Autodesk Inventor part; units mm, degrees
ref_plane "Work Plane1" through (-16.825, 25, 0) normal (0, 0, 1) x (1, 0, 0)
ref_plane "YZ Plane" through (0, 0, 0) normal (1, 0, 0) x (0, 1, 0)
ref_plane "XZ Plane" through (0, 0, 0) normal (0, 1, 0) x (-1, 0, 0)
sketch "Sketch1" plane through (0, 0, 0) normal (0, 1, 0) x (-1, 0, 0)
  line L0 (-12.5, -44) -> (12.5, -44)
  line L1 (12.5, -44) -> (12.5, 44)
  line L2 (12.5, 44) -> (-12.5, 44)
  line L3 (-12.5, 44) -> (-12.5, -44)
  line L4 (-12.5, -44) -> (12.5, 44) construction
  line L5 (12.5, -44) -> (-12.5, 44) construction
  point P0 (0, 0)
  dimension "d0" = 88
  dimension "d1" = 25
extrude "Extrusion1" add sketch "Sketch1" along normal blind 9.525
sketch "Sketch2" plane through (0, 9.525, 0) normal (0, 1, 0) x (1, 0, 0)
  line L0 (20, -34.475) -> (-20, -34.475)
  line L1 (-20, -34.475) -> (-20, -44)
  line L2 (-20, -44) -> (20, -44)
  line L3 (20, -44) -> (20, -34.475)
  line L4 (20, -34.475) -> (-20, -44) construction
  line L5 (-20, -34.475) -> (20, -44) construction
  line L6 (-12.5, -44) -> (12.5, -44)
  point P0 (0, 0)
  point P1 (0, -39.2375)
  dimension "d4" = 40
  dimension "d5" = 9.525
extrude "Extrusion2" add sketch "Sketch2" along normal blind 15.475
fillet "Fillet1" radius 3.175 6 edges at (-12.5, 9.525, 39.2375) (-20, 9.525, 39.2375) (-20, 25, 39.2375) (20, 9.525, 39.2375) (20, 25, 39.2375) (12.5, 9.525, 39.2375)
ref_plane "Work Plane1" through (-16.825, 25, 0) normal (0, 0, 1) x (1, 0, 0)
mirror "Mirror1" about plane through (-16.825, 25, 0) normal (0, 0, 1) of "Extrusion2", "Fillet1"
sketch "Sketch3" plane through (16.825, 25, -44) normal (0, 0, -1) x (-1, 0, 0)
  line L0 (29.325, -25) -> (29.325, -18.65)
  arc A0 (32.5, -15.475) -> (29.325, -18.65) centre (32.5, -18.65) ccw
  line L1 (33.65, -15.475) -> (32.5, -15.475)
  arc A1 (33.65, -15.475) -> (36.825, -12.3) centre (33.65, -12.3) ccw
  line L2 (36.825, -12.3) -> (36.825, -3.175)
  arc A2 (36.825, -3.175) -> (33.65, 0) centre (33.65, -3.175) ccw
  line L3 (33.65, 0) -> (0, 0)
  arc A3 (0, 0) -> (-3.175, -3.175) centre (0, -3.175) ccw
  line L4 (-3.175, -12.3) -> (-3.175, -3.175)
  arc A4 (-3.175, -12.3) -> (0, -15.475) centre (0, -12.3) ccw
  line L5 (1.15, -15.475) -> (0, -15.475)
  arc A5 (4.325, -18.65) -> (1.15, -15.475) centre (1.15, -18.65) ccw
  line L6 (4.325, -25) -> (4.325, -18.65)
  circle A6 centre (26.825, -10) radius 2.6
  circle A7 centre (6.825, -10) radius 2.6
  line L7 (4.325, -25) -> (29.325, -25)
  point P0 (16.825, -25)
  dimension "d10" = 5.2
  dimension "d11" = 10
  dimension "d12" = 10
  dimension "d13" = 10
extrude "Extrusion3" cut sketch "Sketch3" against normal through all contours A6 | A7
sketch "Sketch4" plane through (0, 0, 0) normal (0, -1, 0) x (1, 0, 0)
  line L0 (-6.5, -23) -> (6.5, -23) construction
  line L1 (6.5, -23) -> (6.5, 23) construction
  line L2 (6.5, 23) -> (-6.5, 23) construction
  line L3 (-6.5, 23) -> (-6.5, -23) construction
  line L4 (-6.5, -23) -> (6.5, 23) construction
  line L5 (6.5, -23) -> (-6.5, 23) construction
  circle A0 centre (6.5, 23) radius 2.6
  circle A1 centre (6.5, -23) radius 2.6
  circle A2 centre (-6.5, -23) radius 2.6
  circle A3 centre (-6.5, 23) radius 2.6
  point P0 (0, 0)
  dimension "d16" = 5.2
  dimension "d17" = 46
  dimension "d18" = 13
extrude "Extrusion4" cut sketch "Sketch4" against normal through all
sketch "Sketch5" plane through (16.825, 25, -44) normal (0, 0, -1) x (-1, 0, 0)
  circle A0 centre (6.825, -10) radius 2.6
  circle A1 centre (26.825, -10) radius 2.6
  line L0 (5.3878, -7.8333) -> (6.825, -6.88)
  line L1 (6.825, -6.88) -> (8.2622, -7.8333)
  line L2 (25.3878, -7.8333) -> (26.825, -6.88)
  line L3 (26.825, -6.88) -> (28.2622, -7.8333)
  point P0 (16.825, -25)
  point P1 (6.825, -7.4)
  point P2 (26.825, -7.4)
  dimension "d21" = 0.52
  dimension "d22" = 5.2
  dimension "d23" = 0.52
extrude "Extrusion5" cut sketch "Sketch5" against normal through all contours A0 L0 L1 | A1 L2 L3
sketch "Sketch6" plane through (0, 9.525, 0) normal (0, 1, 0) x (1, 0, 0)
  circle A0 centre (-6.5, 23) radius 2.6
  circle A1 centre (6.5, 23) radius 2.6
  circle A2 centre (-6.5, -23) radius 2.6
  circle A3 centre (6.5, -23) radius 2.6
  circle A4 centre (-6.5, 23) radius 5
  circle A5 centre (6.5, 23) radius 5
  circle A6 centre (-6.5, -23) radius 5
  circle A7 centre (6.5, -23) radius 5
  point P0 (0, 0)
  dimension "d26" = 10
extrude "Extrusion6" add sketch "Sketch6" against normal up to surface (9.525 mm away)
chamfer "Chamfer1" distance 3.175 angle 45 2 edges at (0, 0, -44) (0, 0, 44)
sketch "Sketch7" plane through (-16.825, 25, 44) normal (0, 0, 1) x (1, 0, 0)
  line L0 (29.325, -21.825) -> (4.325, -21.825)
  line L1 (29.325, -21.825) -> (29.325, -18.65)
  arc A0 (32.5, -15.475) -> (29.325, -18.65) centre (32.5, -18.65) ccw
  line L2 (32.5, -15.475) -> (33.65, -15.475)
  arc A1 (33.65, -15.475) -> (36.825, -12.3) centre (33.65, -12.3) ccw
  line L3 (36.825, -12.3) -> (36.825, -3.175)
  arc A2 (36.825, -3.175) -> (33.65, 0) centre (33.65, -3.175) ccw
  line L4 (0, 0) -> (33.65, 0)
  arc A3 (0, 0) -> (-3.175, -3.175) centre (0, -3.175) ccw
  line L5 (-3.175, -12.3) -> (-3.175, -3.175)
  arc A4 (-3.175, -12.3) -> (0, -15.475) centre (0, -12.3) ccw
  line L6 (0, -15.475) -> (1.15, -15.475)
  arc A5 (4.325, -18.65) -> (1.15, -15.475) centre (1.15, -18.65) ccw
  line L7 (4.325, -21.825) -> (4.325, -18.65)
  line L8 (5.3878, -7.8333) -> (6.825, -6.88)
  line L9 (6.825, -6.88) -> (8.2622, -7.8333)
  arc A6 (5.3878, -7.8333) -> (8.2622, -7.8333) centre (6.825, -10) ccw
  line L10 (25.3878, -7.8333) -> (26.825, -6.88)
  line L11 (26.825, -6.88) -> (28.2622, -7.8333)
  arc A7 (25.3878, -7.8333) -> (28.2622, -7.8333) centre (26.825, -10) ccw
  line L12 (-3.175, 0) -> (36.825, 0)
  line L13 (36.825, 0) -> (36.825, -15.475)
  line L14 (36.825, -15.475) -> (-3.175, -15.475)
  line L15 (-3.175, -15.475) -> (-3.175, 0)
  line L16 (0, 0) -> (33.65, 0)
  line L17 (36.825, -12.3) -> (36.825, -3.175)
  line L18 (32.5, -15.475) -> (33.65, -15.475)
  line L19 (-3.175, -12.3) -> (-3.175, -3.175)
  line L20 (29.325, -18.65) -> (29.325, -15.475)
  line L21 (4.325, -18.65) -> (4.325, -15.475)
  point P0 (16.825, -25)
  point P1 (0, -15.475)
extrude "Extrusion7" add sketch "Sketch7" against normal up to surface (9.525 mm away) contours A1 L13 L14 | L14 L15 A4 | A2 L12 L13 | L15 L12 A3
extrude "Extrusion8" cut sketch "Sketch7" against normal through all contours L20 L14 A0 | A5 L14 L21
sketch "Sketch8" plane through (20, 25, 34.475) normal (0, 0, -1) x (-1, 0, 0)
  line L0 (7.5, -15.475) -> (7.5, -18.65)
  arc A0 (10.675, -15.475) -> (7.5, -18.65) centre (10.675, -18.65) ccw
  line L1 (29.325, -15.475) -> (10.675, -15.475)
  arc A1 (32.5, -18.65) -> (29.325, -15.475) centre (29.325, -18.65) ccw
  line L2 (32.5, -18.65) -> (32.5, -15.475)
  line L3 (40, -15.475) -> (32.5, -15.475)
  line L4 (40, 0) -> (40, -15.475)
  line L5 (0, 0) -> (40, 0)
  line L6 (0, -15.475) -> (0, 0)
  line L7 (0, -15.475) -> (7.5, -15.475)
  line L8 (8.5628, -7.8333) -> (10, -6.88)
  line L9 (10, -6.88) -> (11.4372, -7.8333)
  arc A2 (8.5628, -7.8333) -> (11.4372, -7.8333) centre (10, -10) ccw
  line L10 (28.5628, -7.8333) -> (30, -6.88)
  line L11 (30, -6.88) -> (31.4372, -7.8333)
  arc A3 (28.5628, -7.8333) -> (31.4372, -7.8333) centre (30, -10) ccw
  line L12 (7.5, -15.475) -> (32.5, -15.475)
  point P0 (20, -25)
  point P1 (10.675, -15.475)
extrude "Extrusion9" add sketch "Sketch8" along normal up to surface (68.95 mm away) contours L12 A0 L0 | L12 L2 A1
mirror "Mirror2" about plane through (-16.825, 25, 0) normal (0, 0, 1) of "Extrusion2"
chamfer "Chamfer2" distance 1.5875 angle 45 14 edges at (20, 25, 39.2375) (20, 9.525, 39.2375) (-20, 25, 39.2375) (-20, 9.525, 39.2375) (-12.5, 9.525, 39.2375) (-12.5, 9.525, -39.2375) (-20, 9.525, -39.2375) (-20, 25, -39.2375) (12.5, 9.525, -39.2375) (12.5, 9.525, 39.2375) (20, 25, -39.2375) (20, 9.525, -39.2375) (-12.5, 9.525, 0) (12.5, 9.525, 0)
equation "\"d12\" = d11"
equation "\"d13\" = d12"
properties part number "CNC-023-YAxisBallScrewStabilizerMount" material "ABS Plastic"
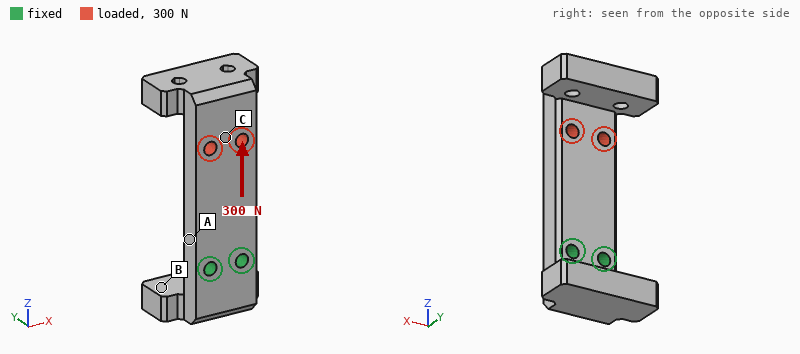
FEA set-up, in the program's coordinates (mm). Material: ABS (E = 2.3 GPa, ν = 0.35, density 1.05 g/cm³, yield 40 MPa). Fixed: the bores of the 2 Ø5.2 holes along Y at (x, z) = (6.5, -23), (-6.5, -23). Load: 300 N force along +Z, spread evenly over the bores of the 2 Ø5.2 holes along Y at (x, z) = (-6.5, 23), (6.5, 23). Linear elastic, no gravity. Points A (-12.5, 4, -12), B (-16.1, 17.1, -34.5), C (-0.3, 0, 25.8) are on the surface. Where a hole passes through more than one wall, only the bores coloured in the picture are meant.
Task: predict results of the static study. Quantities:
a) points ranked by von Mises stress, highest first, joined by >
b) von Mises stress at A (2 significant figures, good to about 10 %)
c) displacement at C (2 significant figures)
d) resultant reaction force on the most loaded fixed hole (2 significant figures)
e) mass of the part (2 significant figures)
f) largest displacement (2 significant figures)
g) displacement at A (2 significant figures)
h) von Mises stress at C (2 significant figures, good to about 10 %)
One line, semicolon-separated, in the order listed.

A > C > B; 1.1 MPa; 25 µm; 150 N; 33 g; 30 µm; 6.4 µm; 0.69 MPa
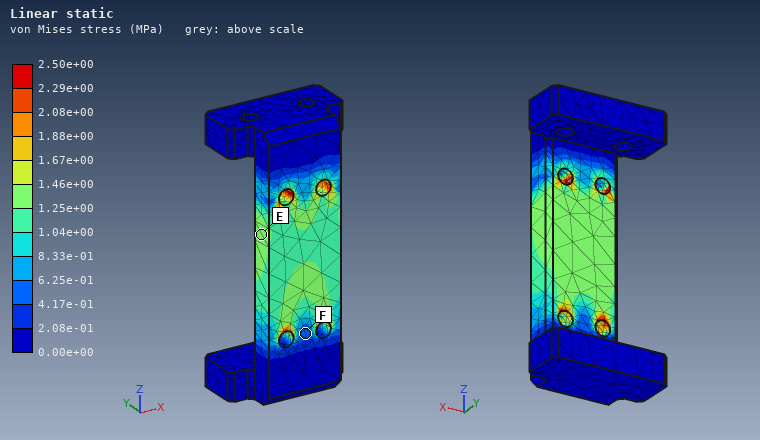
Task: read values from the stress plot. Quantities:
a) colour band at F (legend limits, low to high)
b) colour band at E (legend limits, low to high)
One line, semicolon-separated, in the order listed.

4.17e-01 to 6.25e-01 MPa; 1.25e+00 to 1.46e+00 MPa
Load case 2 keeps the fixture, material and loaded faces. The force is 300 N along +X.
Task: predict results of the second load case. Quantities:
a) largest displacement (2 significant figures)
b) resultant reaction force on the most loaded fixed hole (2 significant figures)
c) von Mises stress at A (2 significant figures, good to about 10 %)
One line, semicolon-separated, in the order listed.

0.72 mm; 860 N; 10 MPa
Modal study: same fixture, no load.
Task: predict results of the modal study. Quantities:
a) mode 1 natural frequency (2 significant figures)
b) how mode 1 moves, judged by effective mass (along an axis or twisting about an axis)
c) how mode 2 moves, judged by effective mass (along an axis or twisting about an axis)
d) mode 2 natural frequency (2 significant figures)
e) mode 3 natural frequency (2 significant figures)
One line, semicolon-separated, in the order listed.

350 Hz; along Y; along X; 730 Hz; 1200 Hz
